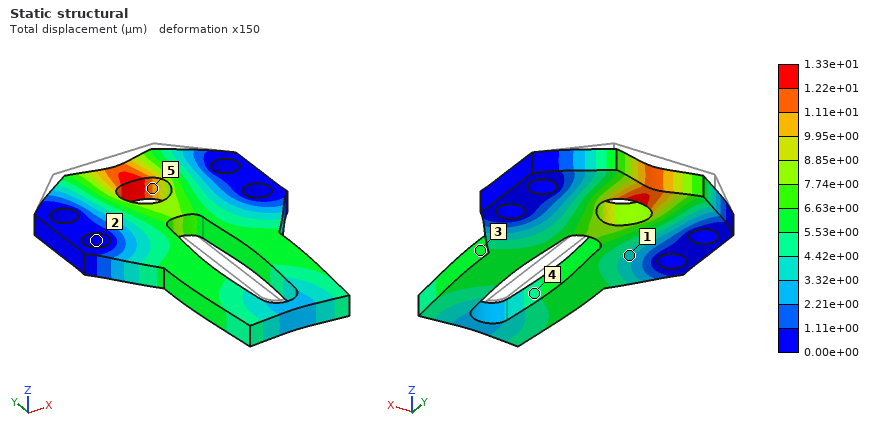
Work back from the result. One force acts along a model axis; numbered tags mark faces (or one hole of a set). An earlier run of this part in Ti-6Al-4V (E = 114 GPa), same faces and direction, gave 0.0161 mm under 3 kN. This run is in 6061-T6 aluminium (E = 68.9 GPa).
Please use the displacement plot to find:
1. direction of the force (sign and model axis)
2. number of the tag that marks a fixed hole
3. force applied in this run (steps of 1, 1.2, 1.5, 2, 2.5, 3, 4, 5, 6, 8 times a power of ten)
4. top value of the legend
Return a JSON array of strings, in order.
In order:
["-Y", "2", "1.5 kN", "1.33e+01 µm"]
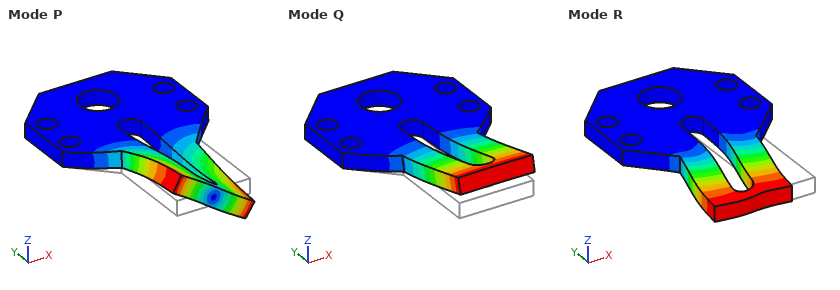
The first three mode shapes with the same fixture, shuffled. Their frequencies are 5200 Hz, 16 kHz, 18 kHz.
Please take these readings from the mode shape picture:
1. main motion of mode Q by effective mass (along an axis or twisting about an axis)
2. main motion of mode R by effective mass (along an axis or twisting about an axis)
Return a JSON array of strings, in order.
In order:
["along Z", "along X"]
